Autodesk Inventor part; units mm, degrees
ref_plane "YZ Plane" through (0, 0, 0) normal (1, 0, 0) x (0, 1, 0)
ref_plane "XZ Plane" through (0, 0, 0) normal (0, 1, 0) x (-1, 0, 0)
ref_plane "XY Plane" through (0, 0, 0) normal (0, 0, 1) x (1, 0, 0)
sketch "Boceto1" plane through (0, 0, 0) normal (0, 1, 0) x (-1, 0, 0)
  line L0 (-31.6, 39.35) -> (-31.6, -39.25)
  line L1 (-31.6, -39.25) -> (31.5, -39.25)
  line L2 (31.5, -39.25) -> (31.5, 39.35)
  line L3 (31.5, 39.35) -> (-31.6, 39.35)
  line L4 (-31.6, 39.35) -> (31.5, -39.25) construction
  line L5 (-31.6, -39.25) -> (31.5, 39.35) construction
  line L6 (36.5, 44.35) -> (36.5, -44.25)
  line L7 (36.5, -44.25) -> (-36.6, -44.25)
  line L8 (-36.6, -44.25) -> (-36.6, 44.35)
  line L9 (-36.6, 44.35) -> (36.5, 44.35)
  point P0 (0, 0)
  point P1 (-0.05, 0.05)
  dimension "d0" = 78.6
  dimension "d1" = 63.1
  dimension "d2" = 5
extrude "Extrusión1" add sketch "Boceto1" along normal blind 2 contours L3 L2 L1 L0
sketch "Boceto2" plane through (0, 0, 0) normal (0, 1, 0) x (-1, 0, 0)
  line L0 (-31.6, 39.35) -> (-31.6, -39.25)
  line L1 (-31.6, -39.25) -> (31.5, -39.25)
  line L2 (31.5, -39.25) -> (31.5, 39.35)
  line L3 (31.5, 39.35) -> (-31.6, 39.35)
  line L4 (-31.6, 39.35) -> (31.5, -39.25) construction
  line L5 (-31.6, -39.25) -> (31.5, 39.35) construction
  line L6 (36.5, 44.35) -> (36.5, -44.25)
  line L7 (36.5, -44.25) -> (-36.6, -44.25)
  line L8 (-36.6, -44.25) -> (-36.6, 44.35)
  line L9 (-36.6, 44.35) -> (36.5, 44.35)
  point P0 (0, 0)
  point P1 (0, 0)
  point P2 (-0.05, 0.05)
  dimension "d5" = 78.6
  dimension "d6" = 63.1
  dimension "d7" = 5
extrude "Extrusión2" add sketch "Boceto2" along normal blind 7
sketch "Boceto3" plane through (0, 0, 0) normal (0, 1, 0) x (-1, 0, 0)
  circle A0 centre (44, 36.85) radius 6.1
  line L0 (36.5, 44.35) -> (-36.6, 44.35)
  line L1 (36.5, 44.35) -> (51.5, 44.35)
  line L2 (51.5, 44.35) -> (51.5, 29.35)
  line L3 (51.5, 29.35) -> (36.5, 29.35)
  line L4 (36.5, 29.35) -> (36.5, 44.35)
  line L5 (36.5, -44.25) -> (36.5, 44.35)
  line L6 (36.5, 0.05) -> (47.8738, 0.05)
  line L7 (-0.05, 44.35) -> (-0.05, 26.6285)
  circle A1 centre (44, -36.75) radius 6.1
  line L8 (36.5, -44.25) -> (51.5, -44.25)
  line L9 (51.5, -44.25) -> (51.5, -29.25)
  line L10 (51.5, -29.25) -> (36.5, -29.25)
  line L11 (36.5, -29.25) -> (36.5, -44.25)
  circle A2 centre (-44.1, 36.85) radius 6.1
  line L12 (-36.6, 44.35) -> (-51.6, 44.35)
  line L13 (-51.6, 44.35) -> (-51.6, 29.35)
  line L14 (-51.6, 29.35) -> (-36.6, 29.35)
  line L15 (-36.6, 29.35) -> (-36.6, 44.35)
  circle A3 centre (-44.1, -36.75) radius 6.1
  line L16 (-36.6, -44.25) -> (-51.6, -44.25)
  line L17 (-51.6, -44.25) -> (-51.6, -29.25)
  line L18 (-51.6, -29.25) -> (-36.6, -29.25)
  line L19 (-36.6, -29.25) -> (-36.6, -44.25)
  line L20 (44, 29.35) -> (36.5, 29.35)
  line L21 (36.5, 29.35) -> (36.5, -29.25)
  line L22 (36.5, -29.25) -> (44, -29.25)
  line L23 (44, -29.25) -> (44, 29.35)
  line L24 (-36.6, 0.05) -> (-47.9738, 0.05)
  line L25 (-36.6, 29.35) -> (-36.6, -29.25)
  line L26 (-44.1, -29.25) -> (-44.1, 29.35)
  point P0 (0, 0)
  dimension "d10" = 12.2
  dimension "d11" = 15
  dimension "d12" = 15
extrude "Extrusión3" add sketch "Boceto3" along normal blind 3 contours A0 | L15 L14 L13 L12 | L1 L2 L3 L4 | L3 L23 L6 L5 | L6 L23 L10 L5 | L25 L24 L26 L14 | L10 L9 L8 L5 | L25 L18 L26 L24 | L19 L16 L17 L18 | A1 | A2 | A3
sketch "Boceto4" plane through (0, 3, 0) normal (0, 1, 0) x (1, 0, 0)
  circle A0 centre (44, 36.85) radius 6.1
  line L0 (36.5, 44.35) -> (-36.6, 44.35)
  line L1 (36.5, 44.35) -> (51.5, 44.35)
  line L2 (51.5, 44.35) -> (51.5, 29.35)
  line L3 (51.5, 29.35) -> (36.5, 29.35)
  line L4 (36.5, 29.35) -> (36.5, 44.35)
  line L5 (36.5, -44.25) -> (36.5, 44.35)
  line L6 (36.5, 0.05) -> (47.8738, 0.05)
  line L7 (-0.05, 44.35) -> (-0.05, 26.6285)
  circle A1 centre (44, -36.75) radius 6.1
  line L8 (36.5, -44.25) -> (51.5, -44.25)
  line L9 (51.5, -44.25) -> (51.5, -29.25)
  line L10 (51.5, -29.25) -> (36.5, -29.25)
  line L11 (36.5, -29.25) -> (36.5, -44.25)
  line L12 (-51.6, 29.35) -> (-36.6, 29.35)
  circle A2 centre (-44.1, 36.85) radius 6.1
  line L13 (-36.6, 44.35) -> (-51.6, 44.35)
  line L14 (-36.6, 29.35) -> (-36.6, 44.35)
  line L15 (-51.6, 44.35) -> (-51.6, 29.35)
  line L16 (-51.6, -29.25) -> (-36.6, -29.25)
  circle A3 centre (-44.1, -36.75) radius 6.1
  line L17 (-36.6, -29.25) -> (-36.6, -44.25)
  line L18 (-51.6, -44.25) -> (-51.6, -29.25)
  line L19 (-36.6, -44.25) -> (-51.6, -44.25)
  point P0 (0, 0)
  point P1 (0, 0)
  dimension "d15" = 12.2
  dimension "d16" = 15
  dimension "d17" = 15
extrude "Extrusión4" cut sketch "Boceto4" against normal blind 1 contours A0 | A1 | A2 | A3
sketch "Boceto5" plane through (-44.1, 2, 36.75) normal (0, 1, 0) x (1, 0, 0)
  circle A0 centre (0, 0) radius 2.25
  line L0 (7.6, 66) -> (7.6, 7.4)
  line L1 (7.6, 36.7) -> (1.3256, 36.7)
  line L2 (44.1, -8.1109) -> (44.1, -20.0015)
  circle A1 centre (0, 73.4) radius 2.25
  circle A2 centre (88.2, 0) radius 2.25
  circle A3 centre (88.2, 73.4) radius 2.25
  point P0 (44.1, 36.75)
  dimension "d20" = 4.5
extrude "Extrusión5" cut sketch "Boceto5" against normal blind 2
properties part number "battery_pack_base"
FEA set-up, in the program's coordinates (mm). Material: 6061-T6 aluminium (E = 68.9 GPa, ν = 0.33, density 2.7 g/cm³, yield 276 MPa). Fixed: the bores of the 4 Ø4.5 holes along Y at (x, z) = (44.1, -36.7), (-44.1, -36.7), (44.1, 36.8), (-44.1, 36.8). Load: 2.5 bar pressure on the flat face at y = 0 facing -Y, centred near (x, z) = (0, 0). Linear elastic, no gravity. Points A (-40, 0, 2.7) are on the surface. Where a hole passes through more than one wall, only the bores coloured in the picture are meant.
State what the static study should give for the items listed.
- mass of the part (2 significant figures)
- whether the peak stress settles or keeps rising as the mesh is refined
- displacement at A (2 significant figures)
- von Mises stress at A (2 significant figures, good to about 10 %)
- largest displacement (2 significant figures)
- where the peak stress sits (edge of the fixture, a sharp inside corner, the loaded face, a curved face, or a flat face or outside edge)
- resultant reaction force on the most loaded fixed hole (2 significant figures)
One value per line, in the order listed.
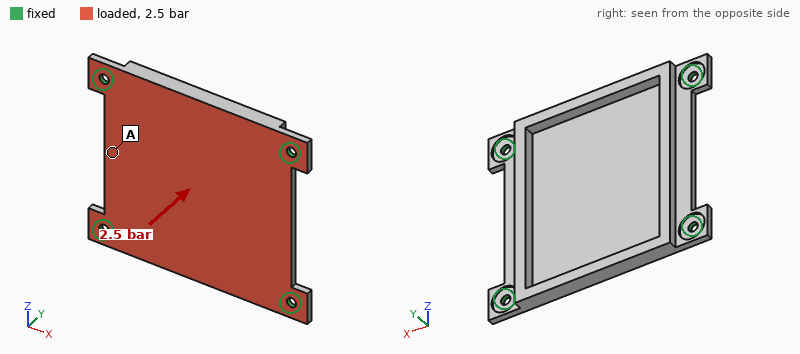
68 g
keeps rising
0.12 mm
25 MPa
0.54 mm
edge of the fixture
860 N
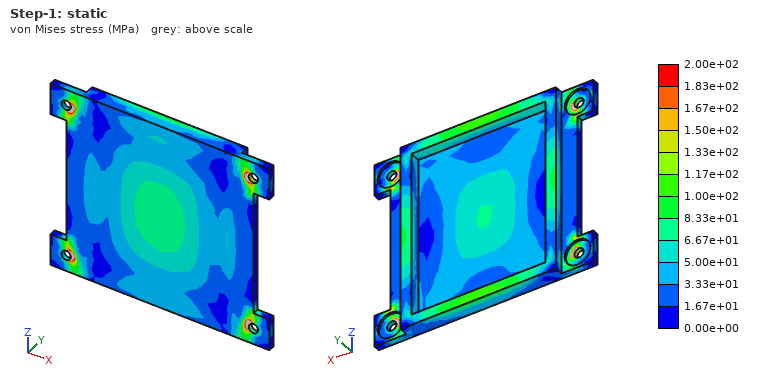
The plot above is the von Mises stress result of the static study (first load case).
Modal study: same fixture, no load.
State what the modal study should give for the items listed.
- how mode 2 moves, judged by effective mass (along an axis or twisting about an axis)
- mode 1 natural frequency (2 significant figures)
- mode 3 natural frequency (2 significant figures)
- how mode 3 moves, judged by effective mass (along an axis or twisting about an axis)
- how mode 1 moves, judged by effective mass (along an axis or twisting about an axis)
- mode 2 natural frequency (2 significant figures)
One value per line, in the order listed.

twisting about X
1800 Hz
3300 Hz
twisting about Z
along Y
2900 Hz
